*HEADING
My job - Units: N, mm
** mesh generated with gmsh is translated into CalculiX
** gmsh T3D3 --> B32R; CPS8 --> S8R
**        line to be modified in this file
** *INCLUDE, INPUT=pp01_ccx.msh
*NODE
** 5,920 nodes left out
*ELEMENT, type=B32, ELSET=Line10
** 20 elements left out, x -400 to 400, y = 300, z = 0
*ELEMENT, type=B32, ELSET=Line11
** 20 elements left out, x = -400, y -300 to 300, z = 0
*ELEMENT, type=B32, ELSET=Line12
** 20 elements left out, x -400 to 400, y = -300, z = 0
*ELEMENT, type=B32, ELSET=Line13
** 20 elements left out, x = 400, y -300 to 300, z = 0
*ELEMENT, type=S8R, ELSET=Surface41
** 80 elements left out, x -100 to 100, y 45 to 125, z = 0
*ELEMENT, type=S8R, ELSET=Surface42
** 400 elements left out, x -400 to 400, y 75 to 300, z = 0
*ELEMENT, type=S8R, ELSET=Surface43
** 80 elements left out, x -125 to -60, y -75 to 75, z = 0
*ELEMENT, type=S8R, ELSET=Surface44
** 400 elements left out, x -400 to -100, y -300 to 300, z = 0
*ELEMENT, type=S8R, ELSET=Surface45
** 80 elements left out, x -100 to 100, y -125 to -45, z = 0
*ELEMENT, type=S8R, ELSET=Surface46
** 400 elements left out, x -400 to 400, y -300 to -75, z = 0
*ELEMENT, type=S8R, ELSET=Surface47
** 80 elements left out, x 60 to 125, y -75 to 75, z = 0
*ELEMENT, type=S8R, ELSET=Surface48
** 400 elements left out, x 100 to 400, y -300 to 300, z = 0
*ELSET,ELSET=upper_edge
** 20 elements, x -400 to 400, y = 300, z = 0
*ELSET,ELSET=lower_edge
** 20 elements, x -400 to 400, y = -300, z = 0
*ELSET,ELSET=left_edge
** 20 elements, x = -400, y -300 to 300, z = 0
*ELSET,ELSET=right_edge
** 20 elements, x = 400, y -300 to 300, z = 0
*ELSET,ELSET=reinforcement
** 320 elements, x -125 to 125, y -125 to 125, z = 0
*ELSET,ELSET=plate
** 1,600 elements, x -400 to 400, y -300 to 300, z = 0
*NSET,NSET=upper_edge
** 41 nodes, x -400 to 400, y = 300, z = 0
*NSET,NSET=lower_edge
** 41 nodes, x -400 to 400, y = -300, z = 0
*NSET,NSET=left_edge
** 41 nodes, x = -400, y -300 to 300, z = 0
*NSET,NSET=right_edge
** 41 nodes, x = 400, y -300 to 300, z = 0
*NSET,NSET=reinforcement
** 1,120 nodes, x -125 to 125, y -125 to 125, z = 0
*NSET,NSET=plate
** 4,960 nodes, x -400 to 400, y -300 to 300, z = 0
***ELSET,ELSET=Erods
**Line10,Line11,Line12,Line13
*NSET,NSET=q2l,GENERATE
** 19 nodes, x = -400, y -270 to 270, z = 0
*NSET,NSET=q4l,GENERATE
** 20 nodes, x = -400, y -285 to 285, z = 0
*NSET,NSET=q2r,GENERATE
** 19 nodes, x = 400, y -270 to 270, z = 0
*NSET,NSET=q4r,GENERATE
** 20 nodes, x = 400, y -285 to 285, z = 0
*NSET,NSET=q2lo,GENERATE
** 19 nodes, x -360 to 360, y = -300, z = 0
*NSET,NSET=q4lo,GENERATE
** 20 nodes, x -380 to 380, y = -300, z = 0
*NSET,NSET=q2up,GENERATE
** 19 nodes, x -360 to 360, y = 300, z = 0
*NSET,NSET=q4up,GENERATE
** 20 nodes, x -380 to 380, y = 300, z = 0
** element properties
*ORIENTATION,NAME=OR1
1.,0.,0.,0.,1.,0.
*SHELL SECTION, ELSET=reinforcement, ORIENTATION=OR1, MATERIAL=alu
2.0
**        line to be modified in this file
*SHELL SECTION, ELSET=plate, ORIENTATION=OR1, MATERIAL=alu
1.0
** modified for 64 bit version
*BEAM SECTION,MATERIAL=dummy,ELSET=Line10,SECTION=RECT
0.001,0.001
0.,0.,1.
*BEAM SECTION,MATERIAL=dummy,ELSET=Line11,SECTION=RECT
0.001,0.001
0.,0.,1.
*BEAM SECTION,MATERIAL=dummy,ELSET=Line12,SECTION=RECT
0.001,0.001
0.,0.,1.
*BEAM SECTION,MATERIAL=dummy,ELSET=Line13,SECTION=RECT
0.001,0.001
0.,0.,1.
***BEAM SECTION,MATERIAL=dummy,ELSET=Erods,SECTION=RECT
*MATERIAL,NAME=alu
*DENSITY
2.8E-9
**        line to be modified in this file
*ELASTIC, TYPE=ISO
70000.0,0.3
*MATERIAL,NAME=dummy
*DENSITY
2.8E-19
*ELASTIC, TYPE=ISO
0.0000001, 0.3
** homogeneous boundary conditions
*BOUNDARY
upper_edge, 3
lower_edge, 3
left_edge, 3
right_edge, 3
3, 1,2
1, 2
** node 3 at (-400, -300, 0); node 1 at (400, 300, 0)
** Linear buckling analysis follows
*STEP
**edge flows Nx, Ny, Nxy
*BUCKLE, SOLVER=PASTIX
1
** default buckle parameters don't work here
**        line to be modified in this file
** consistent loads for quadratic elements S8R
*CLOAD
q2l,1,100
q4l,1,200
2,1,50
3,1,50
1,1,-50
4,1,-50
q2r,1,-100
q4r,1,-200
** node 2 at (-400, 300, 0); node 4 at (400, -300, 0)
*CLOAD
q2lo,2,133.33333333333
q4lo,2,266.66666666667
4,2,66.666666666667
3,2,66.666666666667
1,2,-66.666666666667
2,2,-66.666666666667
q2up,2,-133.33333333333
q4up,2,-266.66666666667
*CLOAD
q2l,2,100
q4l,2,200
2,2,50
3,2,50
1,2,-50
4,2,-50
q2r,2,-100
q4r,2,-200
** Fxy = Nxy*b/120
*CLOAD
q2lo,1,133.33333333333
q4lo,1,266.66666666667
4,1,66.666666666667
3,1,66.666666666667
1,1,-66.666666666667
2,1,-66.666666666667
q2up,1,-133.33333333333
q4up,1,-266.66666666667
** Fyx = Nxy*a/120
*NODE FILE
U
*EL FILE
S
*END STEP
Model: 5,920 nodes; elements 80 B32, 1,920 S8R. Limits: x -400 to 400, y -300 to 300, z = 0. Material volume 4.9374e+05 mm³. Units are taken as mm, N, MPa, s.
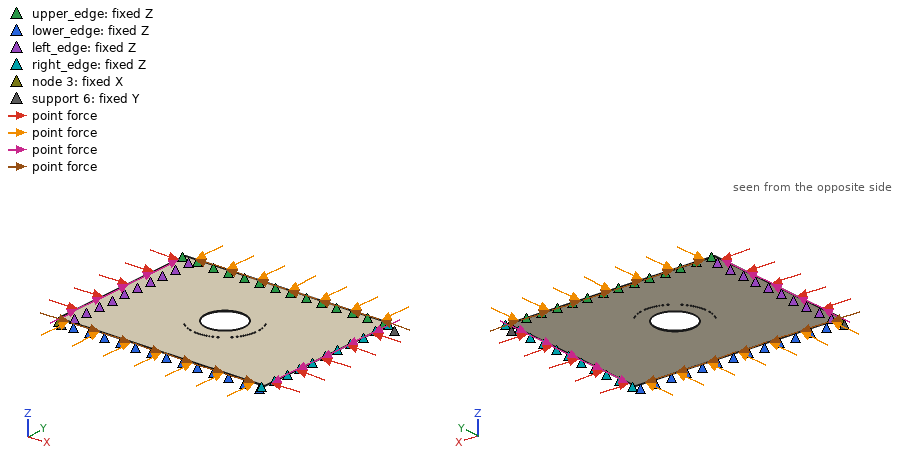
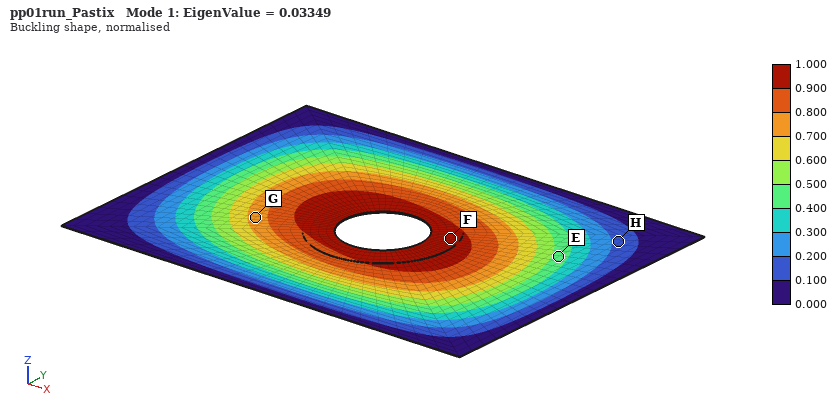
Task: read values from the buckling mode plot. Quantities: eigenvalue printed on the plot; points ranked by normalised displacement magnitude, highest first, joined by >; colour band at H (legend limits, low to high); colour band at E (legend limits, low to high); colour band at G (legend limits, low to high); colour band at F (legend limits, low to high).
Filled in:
0.03349
F > G > E > H
0.100 to 0.200
0.400 to 0.500
0.700 to 0.800
0.900 to 1.000
